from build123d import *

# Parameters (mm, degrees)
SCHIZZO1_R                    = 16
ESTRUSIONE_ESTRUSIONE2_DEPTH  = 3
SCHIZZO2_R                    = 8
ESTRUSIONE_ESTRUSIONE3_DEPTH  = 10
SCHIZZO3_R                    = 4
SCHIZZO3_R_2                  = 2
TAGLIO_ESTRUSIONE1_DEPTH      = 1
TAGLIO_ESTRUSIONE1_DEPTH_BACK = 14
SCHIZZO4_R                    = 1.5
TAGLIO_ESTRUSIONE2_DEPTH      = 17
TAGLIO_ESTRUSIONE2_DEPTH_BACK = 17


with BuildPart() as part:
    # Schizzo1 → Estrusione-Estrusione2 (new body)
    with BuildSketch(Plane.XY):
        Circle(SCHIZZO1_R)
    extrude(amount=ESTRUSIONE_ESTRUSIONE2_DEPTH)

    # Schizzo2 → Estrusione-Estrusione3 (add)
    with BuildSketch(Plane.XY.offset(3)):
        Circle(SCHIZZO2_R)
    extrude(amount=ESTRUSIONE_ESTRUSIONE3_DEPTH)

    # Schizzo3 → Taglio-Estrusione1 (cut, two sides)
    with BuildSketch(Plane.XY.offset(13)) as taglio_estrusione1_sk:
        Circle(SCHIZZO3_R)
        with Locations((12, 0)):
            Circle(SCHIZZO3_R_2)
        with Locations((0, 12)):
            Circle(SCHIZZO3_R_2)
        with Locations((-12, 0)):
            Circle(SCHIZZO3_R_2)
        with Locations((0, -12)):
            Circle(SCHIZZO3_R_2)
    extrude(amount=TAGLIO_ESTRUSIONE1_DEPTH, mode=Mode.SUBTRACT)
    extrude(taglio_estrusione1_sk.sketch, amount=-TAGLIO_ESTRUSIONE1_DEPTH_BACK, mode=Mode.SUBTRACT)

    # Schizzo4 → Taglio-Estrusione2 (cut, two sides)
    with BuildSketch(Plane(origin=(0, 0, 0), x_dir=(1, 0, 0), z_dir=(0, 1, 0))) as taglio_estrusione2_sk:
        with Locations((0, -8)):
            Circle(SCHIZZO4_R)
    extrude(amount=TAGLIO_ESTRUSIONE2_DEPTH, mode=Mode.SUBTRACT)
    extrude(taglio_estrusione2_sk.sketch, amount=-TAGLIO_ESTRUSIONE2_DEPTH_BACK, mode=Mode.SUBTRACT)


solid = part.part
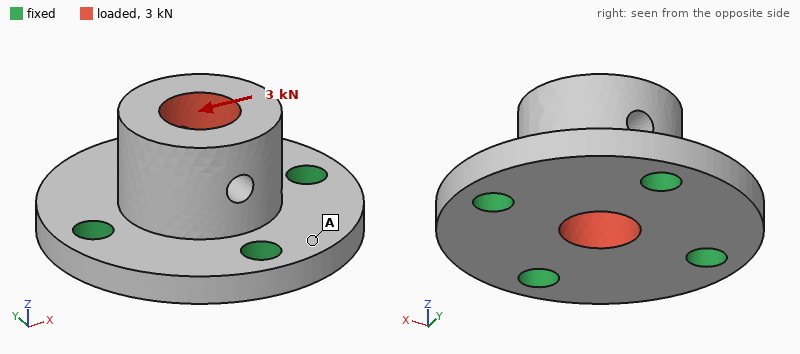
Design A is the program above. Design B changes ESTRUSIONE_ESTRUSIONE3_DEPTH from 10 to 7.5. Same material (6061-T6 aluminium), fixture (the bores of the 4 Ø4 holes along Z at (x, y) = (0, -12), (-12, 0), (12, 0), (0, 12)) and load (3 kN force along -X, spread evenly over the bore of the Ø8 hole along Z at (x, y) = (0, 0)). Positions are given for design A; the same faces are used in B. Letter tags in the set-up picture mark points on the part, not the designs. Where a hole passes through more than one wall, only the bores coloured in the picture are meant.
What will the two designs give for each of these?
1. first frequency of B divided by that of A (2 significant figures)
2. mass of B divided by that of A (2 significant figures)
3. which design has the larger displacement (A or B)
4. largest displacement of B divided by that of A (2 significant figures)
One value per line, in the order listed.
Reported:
1.3
0.89
A
0.66
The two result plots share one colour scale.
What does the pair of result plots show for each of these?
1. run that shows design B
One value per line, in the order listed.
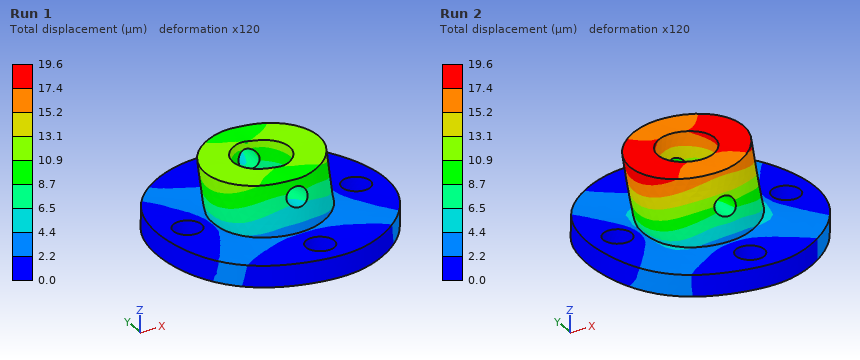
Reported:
Run 1
